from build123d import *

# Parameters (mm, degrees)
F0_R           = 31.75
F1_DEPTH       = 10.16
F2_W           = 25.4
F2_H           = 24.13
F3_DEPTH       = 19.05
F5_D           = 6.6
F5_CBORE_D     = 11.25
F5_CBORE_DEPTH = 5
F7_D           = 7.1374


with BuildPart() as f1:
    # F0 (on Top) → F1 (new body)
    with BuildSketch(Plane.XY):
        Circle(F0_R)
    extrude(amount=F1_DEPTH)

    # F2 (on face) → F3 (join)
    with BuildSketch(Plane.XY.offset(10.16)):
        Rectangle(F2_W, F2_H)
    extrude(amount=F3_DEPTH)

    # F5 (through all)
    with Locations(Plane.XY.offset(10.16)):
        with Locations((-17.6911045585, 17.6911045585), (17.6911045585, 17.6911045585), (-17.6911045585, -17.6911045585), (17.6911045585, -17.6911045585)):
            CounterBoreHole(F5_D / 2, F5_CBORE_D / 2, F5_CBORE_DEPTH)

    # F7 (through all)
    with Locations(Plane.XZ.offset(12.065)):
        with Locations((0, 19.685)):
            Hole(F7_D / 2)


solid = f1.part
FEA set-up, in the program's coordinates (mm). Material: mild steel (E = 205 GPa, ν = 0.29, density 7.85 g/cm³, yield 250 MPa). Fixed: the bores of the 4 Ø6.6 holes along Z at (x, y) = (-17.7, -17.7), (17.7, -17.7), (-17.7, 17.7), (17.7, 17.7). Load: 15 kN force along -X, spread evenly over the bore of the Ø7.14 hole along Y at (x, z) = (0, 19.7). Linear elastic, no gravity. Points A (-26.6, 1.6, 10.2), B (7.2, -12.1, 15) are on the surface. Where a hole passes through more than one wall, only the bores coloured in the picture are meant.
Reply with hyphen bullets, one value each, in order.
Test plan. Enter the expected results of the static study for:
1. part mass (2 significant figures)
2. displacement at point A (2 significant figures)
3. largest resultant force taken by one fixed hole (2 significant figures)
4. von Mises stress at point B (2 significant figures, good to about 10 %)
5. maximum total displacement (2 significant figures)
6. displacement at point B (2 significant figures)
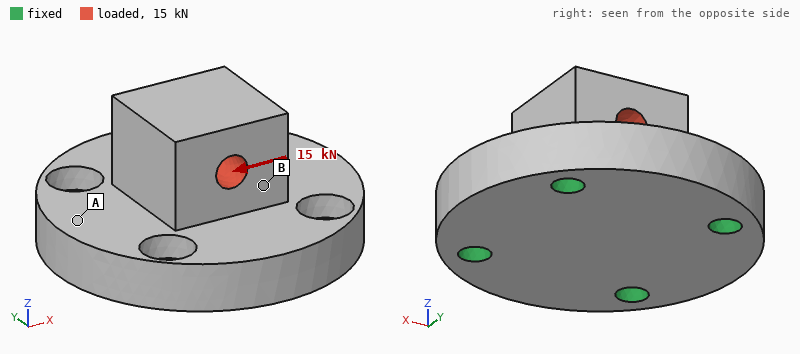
- 320 g
- 6.5 µm
- 5.6 kN
- 54 MPa
- 21 µm
- 8.8 µm
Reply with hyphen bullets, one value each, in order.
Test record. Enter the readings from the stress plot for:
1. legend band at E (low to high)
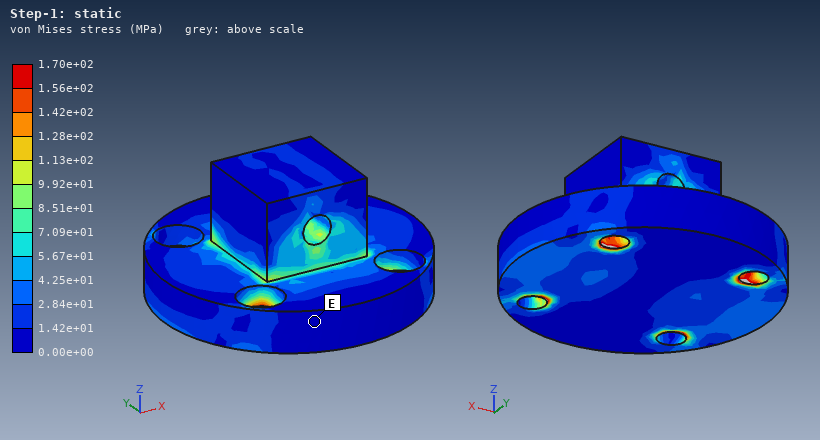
- 0.00e+00 to 1.42e+01 MPa
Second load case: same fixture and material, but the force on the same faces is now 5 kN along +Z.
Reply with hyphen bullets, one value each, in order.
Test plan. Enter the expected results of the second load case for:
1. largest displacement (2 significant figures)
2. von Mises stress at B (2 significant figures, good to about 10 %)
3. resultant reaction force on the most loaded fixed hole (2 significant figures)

- 3.3 µm
- 12 MPa
- 1.5 kN
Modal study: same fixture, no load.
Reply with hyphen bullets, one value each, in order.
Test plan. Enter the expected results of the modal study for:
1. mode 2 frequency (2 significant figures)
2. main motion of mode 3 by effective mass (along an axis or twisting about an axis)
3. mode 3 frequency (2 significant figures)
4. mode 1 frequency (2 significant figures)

- 15 kHz
- along Z
- 17 kHz
- 15 kHz
